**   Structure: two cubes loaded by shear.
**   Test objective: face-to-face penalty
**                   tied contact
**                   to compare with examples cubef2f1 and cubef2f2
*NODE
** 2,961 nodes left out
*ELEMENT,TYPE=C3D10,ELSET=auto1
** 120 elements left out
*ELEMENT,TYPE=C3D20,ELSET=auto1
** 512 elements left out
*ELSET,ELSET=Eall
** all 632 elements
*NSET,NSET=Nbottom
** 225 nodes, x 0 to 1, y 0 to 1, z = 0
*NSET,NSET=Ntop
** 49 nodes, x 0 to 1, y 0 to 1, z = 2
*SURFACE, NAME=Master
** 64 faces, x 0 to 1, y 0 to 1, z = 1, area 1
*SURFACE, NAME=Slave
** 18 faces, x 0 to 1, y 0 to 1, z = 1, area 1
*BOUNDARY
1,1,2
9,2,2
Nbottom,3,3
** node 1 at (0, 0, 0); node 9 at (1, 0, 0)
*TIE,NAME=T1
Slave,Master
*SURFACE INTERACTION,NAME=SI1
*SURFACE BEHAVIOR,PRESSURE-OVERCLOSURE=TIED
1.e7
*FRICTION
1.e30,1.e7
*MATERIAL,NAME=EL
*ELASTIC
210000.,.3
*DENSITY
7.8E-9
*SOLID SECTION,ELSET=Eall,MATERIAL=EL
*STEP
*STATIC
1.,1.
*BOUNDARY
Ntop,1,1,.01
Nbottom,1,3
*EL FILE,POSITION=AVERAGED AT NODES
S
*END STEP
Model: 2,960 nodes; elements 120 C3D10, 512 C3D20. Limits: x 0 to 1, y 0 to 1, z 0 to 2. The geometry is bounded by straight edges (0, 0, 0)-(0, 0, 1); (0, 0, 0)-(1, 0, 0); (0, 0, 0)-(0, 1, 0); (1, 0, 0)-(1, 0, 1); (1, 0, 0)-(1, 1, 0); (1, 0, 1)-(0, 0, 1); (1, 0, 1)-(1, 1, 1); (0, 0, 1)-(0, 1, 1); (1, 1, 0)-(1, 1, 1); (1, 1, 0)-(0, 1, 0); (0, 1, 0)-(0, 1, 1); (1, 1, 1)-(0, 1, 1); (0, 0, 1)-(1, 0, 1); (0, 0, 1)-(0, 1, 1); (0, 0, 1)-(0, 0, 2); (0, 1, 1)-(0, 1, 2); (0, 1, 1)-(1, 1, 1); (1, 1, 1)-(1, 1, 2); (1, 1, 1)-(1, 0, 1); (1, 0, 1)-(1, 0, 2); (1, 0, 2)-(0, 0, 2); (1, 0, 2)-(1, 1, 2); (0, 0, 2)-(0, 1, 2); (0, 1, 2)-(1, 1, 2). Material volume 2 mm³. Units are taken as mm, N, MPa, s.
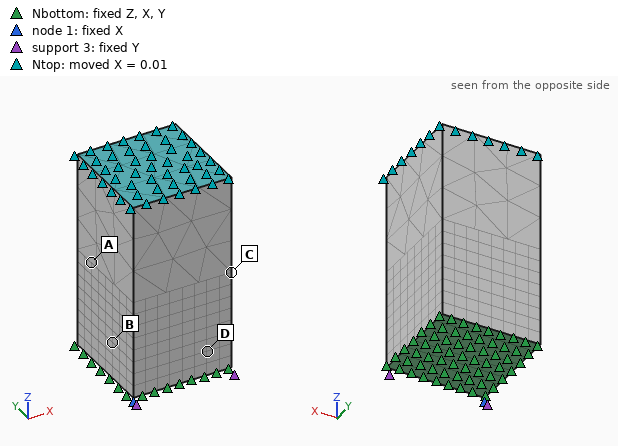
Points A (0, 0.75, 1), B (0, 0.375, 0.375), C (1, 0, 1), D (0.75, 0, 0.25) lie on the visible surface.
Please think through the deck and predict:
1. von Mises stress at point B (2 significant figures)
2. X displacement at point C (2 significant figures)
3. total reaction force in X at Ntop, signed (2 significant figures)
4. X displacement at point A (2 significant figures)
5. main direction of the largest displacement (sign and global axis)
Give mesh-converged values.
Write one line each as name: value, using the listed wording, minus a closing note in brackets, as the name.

von Mises stress at point B: 530 MPa
X displacement at point C: 0.0033 mm
total reaction force in X at Ntop, signed: 55 N
X displacement at point A: 0.0034 mm
main direction of the largest displacement: +X
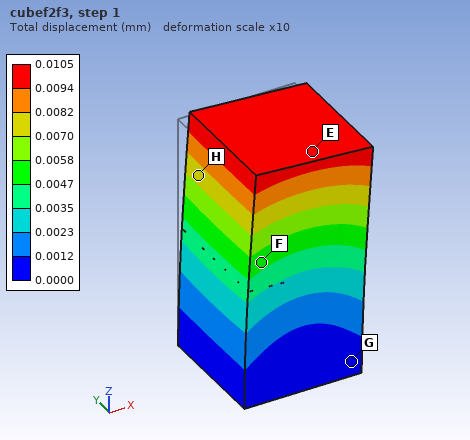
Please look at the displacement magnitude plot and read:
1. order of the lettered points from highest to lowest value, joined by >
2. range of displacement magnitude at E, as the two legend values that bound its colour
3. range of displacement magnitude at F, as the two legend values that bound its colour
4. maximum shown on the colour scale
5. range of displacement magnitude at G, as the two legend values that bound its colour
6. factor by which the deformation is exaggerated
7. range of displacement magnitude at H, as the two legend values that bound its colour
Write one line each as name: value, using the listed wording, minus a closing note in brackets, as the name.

order of the lettered points from highest to lowest value, joined by >: E > H > F > G
range of displacement magnitude at E, as the two legend values that bound its colour: 0.0094 to 0.0105 mm
range of displacement magnitude at F, as the two legend values that bound its colour: 0.0047 to 0.0058 mm
maximum shown on the colour scale: 0.0105 mm
range of displacement magnitude at G, as the two legend values that bound its colour: 0.0000 to 0.0012 mm
factor by which the deformation is exaggerated: 10
range of displacement magnitude at H, as the two legend values that bound its colour: 0.0070 to 0.0082 mm
